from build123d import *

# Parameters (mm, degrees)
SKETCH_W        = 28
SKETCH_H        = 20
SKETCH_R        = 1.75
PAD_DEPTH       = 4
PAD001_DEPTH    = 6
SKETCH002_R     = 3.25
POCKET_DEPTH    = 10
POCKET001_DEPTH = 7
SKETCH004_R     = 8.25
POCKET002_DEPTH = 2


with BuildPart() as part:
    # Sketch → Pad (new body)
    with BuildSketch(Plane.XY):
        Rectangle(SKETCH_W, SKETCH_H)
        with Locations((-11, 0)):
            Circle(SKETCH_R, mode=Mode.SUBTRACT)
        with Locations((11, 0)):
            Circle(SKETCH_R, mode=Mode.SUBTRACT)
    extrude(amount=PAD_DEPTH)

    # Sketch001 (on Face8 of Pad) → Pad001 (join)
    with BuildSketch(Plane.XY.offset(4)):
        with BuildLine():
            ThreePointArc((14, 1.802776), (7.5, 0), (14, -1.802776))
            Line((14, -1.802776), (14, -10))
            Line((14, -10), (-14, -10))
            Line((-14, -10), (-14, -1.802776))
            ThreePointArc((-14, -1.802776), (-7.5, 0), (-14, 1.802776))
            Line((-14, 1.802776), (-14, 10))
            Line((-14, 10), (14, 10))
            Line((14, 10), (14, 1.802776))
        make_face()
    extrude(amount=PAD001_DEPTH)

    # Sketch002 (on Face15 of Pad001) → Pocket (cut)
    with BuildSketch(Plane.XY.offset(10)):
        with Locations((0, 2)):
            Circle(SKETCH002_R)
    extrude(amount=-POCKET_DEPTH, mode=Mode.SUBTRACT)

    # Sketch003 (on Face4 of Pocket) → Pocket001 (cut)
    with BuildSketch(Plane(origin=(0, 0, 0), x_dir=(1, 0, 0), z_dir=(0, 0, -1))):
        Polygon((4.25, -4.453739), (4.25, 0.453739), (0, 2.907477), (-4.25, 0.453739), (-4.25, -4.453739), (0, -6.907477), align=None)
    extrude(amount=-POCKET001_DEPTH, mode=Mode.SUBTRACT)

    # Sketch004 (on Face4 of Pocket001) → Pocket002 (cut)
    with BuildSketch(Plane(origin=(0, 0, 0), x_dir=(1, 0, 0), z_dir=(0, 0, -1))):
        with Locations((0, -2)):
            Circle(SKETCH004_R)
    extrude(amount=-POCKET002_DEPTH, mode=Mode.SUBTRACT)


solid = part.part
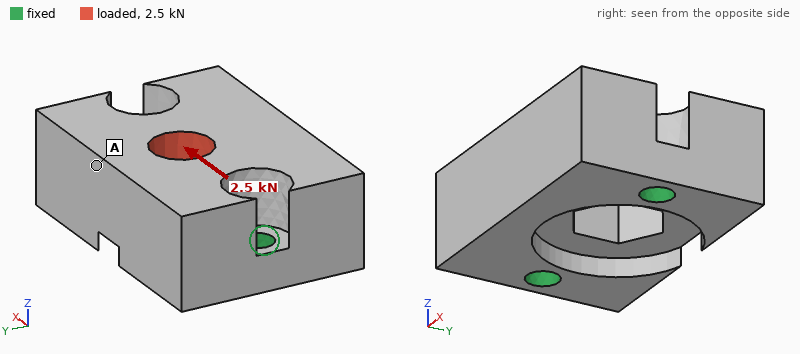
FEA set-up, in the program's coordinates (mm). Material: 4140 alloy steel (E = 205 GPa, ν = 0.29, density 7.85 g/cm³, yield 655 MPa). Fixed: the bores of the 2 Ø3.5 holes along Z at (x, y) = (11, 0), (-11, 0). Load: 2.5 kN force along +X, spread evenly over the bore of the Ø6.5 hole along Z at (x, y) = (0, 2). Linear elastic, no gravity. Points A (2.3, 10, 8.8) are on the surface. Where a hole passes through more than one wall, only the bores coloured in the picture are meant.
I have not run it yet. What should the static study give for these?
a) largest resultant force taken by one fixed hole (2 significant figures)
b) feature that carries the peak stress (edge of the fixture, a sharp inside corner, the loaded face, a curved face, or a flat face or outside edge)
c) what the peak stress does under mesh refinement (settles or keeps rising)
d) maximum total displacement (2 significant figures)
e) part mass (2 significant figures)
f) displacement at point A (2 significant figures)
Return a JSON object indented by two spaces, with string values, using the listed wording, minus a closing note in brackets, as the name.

{
  "largest resultant force taken by one fixed hole": "1.4 kN",
  "feature that carries the peak stress": "edge of the fixture",
  "what the peak stress does under mesh refinement": "keeps rising",
  "maximum total displacement": "3.8 µm",
  "part mass": "33 g",
  "displacement at point A": "2.4 µm"
}
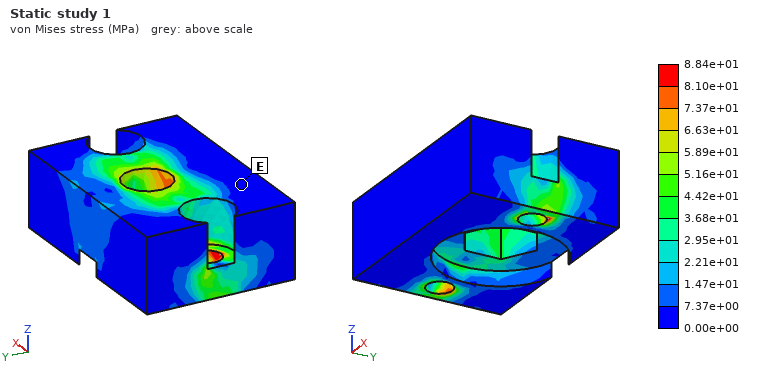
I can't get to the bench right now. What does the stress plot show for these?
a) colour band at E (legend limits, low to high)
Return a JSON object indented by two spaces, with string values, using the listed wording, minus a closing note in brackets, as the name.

{
  "colour band at E": "0.00e+00 to 7.37e+00 MPa"
}
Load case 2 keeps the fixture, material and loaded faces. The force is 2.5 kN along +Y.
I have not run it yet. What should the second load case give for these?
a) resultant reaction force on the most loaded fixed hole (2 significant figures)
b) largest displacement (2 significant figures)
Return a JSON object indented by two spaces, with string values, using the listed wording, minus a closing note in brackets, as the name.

{
  "resultant reaction force on the most loaded fixed hole": "1.3 kN",
  "largest displacement": "18 µm"
}
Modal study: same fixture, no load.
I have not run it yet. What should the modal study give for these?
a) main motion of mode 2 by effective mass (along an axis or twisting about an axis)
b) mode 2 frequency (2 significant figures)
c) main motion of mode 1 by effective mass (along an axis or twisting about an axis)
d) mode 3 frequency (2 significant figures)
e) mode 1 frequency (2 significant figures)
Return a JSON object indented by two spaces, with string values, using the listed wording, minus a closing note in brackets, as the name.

{
  "main motion of mode 2 by effective mass": "along Z",
  "mode 2 frequency": "30 kHz",
  "main motion of mode 1 by effective mass": "along Y",
  "mode 3 frequency": "32 kHz",
  "mode 1 frequency": "14 kHz"
}
